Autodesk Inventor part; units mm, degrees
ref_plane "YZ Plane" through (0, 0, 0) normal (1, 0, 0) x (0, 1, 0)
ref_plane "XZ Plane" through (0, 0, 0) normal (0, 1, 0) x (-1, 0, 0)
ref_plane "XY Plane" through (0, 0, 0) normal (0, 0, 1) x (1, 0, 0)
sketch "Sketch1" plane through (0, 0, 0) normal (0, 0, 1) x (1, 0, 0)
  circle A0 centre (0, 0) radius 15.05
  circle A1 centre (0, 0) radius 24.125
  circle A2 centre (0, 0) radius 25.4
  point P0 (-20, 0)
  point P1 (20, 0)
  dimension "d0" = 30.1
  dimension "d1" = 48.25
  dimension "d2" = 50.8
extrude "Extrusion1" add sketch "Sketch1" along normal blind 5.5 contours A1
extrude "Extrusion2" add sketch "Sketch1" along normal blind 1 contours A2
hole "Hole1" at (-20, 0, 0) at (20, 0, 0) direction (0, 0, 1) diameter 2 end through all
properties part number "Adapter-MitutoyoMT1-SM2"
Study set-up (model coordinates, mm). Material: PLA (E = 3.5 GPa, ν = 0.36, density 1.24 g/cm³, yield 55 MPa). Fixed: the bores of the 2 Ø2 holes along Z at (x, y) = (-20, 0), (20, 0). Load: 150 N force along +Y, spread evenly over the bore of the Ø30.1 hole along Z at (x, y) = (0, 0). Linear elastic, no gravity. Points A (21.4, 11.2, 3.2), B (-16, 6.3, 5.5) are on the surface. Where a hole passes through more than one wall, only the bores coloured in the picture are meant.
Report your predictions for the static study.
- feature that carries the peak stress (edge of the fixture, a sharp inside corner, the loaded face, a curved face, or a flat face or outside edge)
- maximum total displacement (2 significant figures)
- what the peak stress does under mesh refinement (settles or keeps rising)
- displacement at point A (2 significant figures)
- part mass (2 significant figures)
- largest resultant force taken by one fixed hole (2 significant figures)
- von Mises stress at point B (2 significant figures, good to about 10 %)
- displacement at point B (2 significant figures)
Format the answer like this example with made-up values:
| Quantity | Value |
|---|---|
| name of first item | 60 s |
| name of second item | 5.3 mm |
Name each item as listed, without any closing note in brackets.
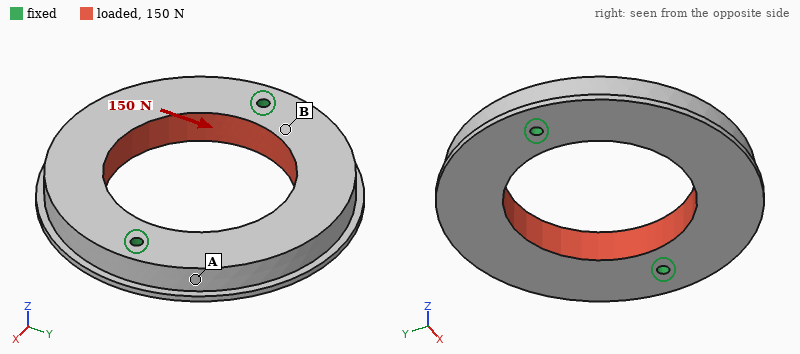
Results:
| Quantity | Value |
|---|---|
| feature that carries the peak stress | edge of the fixture |
| maximum total displacement | 8.7 µm |
| what the peak stress does under mesh refinement | keeps rising |
| displacement at point A | 1.9 µm |
| part mass | 7.8 g |
| largest resultant force taken by one fixed hole | 75 N |
| von Mises stress at point B | 1.0 MPa |
| displacement at point B | 2.9 µm |
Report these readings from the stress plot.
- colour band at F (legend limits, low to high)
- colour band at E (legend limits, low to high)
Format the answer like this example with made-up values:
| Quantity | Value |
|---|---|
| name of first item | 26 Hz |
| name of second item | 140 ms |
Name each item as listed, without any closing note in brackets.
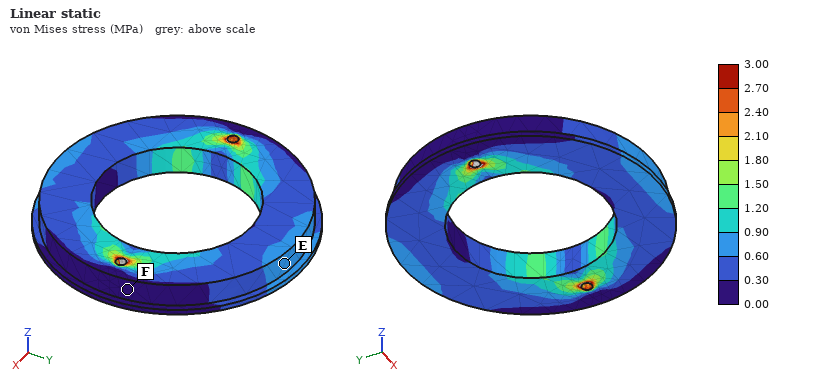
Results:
| Quantity | Value |
|---|---|
| colour band at F | 0.00 to 0.30 MPa |
| colour band at E | 0.60 to 0.90 MPa |
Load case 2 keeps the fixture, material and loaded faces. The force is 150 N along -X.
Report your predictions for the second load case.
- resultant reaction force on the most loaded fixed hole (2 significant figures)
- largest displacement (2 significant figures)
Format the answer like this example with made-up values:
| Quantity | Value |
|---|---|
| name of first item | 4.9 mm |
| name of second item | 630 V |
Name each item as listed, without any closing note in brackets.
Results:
| Quantity | Value |
|---|---|
| resultant reaction force on the most loaded fixed hole | 75 N |
| largest displacement | 16 µm |
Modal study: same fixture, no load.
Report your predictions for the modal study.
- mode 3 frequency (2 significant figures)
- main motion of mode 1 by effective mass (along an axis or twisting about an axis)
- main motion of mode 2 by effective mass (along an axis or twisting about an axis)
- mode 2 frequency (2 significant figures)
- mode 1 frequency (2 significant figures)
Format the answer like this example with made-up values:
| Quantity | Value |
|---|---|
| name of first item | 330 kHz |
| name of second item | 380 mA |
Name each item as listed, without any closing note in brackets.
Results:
| Quantity | Value |
|---|---|
| mode 3 frequency | 4400 Hz |
| main motion of mode 1 by effective mass | twisting about X |
| main motion of mode 2 by effective mass | along Z |
| mode 2 frequency | 1900 Hz |
| mode 1 frequency | 1700 Hz |
